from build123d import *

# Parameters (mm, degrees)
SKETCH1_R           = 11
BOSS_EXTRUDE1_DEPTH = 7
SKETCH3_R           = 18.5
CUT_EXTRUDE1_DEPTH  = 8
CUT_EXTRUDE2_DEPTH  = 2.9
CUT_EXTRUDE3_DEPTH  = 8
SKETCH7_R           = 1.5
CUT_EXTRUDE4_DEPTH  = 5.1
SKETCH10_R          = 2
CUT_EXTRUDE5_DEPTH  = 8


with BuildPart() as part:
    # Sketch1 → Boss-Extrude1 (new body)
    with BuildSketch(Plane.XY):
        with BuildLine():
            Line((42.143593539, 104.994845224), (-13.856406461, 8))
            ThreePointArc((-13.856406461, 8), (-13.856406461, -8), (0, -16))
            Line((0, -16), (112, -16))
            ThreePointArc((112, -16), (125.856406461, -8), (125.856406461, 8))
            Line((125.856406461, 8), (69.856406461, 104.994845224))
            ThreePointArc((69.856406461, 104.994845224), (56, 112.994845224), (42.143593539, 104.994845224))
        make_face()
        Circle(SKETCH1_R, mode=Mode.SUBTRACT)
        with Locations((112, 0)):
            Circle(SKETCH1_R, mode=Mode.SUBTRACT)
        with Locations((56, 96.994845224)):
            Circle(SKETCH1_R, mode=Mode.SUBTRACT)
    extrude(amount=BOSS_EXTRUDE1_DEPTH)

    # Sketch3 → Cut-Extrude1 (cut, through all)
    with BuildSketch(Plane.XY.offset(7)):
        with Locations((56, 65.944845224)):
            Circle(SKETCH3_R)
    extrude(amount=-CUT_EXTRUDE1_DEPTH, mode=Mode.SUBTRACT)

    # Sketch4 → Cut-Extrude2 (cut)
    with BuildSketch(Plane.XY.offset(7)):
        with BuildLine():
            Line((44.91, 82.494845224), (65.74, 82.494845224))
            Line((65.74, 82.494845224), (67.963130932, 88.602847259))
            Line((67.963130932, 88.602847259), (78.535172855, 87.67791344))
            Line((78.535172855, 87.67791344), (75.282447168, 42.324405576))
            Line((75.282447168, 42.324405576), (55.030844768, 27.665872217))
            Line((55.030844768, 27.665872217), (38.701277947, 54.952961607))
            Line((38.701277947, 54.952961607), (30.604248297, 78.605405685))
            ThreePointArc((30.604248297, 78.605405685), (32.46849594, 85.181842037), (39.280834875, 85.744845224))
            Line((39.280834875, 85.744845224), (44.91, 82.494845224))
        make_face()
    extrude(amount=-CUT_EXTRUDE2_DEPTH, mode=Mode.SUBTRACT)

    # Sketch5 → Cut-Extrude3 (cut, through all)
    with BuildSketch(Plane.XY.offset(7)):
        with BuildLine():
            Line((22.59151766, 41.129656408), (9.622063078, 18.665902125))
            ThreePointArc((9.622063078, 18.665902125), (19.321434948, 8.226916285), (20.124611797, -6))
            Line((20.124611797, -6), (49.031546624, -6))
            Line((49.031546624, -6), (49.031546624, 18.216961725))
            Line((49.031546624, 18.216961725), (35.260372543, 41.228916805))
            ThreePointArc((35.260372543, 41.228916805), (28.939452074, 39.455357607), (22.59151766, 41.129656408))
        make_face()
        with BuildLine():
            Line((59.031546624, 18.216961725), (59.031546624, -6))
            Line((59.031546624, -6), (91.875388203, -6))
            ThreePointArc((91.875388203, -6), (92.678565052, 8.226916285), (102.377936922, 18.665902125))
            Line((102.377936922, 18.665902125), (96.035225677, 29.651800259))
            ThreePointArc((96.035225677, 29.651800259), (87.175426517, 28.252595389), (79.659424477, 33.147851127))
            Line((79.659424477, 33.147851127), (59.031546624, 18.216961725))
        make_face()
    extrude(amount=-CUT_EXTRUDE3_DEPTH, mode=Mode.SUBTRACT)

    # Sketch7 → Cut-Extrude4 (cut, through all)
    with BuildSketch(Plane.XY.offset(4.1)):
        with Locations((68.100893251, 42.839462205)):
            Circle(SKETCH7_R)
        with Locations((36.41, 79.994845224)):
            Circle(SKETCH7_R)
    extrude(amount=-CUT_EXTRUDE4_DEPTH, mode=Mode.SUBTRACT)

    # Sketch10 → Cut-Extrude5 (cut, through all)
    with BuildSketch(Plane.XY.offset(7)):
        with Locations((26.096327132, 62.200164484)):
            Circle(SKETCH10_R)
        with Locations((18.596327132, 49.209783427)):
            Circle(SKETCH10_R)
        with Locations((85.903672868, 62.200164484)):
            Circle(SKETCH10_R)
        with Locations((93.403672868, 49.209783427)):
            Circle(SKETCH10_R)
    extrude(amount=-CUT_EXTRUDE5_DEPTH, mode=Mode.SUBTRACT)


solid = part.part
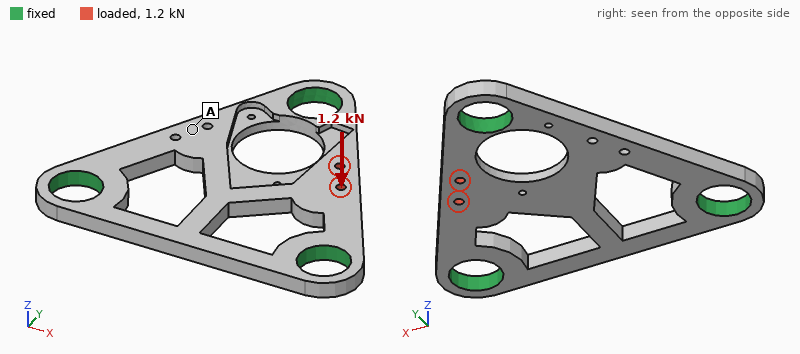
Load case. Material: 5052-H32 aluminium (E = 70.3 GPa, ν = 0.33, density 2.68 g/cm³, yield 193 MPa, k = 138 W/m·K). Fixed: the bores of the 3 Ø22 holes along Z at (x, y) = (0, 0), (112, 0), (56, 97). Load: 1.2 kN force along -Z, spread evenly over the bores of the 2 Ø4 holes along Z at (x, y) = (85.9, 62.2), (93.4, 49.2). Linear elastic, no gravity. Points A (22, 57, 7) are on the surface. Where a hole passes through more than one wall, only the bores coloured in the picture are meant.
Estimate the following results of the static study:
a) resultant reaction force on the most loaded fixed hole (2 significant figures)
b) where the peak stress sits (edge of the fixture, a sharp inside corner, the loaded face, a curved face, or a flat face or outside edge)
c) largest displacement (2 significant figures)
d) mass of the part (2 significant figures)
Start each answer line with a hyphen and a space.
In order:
- 650 N
- the loaded face
- 0.17 mm
- 120 g
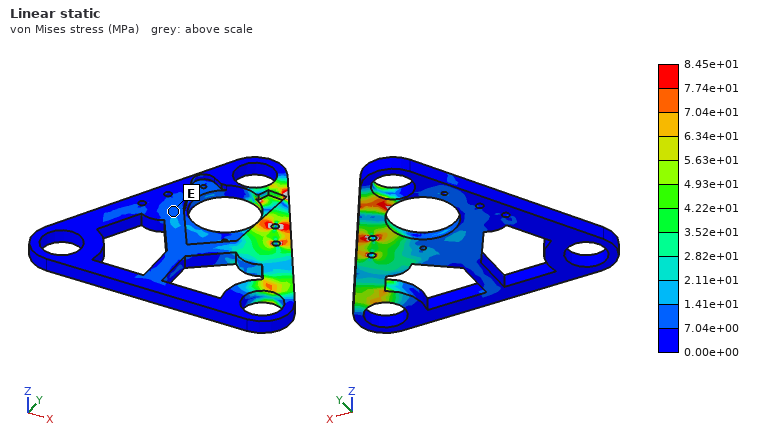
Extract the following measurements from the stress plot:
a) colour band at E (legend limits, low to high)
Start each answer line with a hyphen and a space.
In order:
- 7.04e+00 to 1.41e+01 MPa
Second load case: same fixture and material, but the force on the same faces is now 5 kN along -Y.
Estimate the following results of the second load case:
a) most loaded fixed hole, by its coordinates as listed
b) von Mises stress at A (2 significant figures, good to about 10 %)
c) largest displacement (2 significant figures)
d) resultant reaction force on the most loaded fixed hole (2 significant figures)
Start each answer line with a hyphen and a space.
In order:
- (112, 0)
- 8.0 MPa
- 40 µm
- 2.5 kN
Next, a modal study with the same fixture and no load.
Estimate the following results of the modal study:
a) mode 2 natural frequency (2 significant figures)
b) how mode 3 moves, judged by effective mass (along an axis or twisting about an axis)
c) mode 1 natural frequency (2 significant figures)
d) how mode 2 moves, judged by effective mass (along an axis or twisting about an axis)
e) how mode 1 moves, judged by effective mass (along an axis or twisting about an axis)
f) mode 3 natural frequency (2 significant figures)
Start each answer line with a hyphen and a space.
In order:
- 3900 Hz
- twisting about X
- 2600 Hz
- twisting about Y
- along Z
- 4100 Hz
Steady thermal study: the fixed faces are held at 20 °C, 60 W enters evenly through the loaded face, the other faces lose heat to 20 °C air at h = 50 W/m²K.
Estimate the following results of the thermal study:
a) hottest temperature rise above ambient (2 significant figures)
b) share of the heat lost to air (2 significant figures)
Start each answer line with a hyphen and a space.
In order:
- 62 K
- 23 %
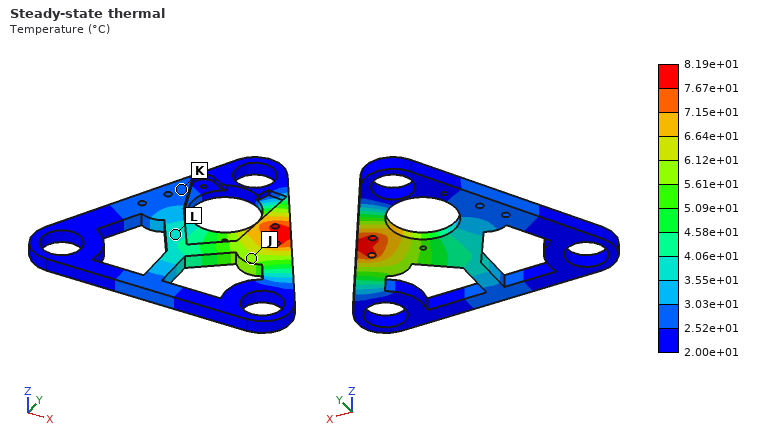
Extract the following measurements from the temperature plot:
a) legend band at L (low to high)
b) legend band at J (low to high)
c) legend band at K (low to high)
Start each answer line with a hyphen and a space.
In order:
- 3.55e+01 to 4.06e+01 °C
- 5.61e+01 to 6.12e+01 °C
- 2.52e+01 to 3.03e+01 °C
